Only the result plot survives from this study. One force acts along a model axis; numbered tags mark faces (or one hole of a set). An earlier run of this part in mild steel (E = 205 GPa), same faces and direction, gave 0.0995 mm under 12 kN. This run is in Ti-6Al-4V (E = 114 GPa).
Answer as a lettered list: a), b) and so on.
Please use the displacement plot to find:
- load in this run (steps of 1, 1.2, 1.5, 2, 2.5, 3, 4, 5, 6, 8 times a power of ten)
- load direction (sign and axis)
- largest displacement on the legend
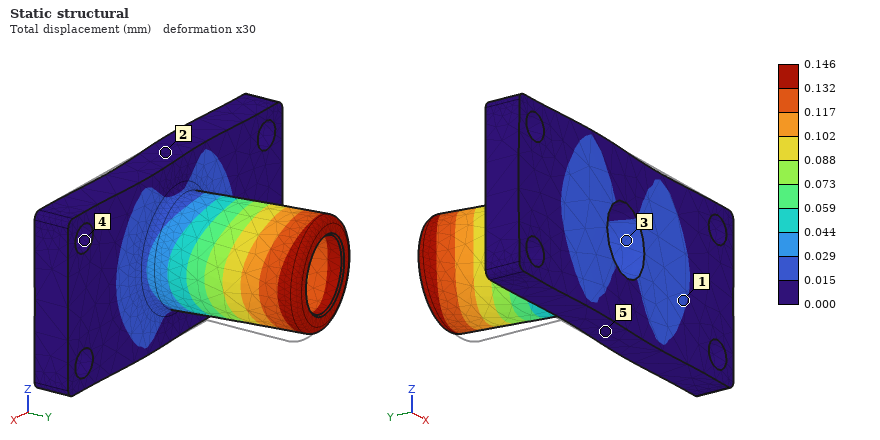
a) 10 kN
b) -X
c) 0.146 mm
